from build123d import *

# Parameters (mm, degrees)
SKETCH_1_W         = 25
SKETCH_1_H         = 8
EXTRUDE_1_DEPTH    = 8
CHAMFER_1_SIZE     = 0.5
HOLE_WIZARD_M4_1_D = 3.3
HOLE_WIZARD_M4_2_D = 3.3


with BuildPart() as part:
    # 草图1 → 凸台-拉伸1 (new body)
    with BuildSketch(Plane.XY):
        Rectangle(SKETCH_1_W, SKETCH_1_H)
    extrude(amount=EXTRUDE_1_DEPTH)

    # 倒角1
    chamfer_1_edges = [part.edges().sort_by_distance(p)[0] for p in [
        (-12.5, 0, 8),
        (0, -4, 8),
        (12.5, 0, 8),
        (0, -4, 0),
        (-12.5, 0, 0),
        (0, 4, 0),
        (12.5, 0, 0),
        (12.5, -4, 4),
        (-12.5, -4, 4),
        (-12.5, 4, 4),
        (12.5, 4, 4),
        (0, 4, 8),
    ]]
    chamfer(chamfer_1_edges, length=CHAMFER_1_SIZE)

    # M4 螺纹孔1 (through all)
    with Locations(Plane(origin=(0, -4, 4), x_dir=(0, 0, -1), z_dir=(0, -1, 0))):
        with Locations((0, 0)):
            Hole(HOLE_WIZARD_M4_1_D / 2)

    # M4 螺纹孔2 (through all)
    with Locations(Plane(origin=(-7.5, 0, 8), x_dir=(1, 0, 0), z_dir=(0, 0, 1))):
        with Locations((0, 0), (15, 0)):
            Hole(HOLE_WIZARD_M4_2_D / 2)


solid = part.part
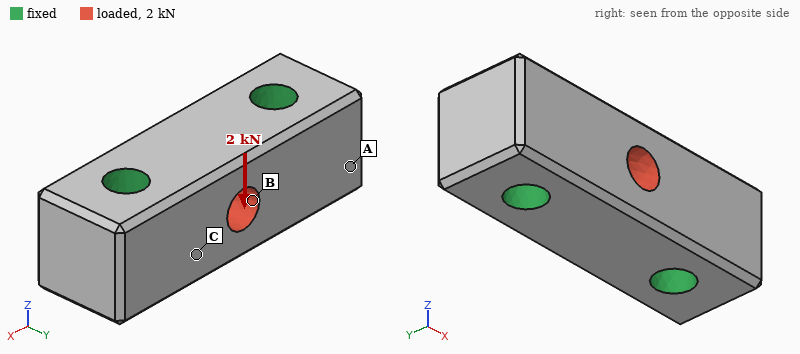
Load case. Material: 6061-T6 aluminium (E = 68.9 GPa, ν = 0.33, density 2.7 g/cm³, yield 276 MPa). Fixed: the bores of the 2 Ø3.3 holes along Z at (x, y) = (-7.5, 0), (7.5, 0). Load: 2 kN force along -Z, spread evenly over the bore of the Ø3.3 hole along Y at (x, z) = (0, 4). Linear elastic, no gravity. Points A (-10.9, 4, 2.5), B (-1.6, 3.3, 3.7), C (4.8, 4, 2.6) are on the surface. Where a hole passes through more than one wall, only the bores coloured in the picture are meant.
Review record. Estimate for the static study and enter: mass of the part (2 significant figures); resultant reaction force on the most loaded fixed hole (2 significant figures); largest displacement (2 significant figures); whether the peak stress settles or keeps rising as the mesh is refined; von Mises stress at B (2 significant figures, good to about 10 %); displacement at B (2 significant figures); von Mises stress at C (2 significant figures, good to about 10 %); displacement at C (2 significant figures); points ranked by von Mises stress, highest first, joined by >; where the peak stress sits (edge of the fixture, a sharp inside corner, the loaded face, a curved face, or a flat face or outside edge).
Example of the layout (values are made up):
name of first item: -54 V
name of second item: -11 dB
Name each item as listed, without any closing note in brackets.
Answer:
mass of the part: 3.7 g
resultant reaction force on the most loaded fixed hole: 1.0 kN
largest displacement: 5.7 µm
whether the peak stress settles or keeps rising as the mesh is refined: keeps rising
von Mises stress at B: 46 MPa
displacement at B: 4.6 µm
von Mises stress at C: 26 MPa
displacement at C: 1.7 µm
points ranked by von Mises stress, highest first, joined by >: B > C > A
where the peak stress sits: edge of the fixture
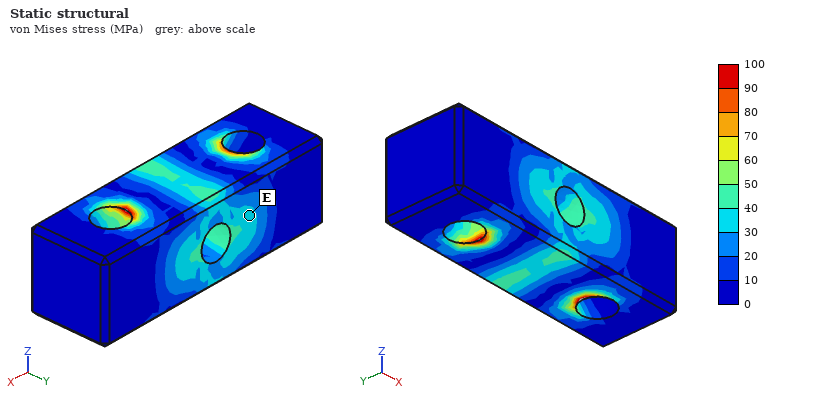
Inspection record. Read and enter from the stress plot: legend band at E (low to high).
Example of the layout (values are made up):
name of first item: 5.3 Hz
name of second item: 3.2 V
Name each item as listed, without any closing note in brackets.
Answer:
legend band at E: 30 to 40 MPa
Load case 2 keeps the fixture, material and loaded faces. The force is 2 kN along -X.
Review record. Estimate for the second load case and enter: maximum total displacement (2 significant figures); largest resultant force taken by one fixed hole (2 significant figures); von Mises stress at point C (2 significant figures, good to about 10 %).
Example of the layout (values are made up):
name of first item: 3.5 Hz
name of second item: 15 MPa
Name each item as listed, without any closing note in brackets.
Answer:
maximum total displacement: 1.9 µm
largest resultant force taken by one fixed hole: 1.0 kN
von Mises stress at point C: 12 MPa
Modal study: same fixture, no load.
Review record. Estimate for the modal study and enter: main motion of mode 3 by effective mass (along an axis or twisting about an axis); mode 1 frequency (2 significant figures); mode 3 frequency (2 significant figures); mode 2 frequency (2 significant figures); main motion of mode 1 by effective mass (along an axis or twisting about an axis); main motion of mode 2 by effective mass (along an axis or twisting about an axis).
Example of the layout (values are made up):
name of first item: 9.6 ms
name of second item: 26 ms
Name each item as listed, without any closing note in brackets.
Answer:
main motion of mode 3 by effective mass: twisting about X
mode 1 frequency: 90 kHz
mode 3 frequency: 110 kHz
mode 2 frequency: 110 kHz
main motion of mode 1 by effective mass: along Y
main motion of mode 2 by effective mass: along Z
